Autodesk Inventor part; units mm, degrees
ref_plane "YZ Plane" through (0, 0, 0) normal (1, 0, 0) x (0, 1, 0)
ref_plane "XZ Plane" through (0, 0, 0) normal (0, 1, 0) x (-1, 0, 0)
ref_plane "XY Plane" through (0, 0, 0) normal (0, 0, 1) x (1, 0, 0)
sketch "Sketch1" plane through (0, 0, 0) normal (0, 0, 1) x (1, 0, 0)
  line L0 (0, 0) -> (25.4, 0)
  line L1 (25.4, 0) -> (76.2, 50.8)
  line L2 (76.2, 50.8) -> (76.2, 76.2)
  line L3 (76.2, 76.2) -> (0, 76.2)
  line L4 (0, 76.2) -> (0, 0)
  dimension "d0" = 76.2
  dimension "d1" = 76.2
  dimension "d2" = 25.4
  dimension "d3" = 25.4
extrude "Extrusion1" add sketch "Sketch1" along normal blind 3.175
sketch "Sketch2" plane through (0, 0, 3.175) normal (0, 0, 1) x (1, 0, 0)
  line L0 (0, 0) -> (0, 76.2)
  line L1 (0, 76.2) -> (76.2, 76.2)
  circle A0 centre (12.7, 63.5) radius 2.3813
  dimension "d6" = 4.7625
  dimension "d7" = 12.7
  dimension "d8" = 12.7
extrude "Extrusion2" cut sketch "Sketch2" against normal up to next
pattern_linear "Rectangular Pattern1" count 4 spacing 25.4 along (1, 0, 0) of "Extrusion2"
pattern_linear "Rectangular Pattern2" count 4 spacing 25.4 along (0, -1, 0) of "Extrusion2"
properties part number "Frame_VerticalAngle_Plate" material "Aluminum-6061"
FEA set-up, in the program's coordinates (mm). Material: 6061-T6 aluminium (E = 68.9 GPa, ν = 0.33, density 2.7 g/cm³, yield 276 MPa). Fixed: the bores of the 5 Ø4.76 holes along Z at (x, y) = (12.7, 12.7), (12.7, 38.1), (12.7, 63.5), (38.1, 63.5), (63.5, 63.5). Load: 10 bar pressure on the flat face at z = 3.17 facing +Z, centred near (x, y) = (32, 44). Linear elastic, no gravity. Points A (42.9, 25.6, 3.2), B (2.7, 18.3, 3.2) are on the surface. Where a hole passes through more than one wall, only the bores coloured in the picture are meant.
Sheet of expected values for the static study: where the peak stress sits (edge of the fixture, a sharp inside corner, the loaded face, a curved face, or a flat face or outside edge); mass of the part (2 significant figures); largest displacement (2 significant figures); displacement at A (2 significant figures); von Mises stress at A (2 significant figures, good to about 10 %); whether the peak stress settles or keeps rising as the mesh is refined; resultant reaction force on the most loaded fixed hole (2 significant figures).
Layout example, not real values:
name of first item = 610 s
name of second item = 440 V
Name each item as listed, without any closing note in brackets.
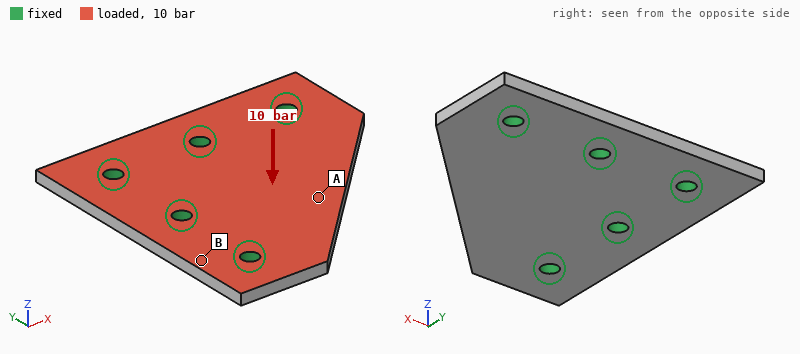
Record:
where the peak stress sits = edge of the fixture
mass of the part = 38 g
largest displacement = 0.41 mm
displacement at A = 0.32 mm
von Mises stress at A = 72 MPa
whether the peak stress settles or keeps rising as the mesh is refined = keeps rising
resultant reaction force on the most loaded fixed hole = 1.0 kN
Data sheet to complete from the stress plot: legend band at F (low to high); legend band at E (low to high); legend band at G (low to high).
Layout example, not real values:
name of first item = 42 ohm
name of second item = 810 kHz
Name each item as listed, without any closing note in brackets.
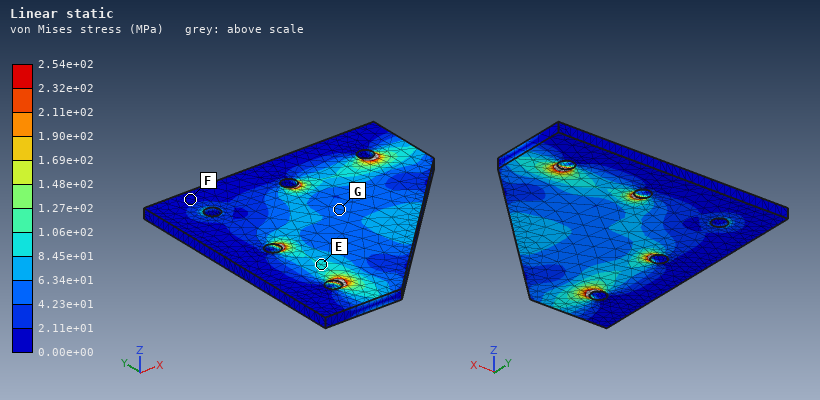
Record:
legend band at F = 0.00e+00 to 2.11e+01 MPa
legend band at E = 8.45e+01 to 1.06e+02 MPa
legend band at G = 4.23e+01 to 6.34e+01 MPa
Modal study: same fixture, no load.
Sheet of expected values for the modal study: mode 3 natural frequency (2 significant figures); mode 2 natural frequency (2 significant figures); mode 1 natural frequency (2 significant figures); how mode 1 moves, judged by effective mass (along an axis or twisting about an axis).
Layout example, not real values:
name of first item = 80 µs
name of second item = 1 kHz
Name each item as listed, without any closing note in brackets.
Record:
mode 3 natural frequency = 11 kHz
mode 2 natural frequency = 7600 Hz
mode 1 natural frequency = 3700 Hz
how mode 1 moves, judged by effective mass = along Z
